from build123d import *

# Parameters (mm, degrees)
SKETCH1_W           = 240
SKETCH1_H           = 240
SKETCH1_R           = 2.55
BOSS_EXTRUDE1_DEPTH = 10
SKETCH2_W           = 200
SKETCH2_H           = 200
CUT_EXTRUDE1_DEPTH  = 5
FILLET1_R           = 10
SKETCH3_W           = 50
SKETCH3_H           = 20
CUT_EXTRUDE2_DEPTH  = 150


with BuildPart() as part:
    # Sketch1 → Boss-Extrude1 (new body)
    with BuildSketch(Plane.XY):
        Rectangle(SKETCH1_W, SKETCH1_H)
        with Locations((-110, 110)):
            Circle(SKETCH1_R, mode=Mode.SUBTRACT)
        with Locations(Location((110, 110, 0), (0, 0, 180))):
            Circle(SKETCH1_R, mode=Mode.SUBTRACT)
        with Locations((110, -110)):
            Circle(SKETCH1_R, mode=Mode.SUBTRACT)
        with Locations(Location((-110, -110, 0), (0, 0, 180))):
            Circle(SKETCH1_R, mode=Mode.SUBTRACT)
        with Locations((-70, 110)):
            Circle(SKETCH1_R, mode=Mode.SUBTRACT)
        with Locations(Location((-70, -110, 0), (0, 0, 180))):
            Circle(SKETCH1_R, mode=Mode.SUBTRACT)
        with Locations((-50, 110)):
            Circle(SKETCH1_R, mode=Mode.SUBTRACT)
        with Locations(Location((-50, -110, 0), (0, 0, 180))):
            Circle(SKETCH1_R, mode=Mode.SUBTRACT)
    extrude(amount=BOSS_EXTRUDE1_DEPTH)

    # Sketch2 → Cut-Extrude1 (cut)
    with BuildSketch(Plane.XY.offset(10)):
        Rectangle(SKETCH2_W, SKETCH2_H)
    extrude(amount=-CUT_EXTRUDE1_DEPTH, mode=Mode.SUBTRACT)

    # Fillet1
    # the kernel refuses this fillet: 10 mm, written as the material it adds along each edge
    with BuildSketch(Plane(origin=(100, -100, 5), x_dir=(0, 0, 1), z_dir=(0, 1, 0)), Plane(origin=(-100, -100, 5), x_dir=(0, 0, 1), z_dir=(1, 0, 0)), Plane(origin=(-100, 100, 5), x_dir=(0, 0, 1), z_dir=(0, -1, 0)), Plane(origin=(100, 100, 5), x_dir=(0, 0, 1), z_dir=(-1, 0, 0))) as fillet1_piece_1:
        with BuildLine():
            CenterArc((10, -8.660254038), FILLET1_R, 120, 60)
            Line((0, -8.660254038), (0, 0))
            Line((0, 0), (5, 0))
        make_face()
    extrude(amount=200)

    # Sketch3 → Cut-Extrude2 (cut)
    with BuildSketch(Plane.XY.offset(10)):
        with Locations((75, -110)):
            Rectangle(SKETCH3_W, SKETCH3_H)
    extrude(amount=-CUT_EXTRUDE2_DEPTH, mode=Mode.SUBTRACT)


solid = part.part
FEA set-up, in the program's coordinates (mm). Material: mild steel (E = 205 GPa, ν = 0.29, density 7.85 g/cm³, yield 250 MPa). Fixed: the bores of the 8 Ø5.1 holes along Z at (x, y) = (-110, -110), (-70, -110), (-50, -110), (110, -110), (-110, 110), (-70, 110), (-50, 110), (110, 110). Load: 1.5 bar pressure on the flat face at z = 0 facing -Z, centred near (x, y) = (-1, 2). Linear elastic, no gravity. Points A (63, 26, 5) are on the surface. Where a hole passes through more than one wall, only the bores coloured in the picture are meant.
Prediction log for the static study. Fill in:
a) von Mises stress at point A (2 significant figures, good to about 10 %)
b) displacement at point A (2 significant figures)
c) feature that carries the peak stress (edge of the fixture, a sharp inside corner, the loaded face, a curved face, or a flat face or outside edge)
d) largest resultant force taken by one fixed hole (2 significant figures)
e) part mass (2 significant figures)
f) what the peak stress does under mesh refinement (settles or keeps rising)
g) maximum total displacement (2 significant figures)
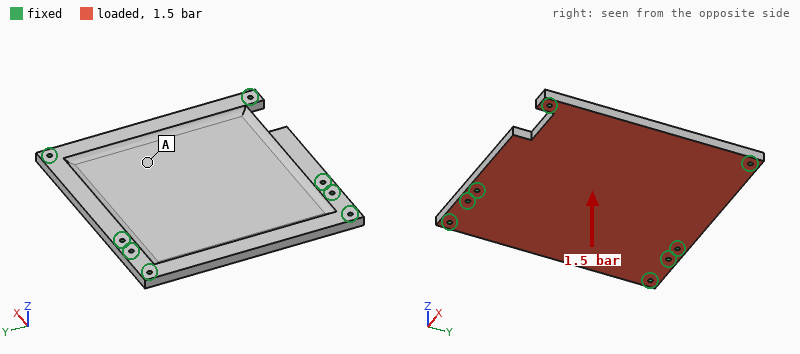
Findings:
25 MPa
0.24 mm
edge of the fixture
3.3 kN
2.9 kg
keeps rising
0.31 mm
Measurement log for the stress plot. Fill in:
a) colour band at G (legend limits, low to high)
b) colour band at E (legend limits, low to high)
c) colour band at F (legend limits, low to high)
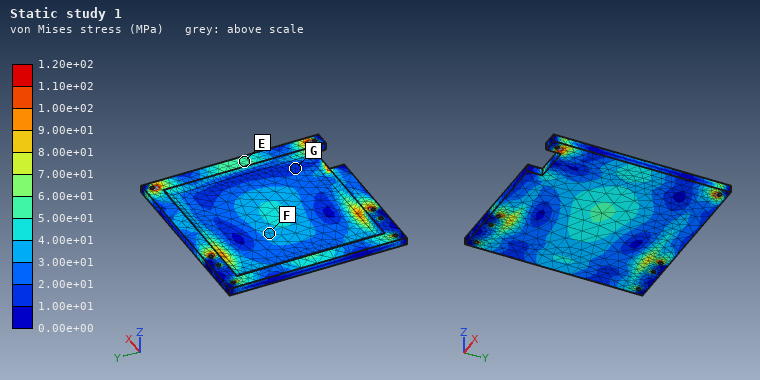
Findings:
1.00e+01 to 2.00e+01 MPa
5.00e+01 to 6.00e+01 MPa
3.00e+01 to 4.00e+01 MPa
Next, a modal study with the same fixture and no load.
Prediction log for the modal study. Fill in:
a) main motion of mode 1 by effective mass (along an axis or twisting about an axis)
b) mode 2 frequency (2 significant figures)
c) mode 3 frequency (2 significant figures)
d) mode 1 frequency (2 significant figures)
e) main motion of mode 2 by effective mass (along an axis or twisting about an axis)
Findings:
along Z
960 Hz
1200 Hz
680 Hz
twisting about Y
